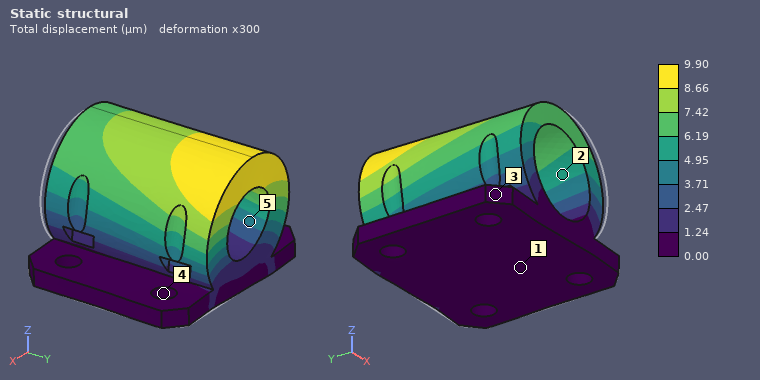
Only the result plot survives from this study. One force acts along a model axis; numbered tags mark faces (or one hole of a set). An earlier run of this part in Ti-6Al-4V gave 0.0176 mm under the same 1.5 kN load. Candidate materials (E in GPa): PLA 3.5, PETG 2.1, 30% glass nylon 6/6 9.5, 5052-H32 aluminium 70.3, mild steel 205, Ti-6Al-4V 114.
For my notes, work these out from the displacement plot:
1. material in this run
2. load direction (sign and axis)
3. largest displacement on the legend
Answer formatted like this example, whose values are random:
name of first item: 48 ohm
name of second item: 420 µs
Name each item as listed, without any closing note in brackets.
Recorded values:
material in this run: mild steel
load direction: -X
largest displacement on the legend: 9.90 µm
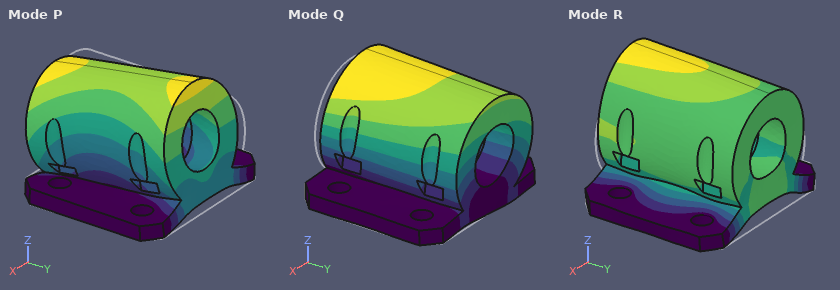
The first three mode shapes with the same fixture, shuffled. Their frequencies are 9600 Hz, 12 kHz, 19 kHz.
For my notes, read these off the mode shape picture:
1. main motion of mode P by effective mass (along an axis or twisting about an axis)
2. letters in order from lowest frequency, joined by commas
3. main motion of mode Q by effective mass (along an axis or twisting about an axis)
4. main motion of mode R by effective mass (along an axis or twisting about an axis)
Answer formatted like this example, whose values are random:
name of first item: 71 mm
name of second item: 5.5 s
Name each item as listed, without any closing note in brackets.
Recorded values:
main motion of mode P by effective mass: along Y
letters in order from lowest frequency, joined by commas: Q, P, R
main motion of mode Q by effective mass: along X
main motion of mode R by effective mass: along Z
